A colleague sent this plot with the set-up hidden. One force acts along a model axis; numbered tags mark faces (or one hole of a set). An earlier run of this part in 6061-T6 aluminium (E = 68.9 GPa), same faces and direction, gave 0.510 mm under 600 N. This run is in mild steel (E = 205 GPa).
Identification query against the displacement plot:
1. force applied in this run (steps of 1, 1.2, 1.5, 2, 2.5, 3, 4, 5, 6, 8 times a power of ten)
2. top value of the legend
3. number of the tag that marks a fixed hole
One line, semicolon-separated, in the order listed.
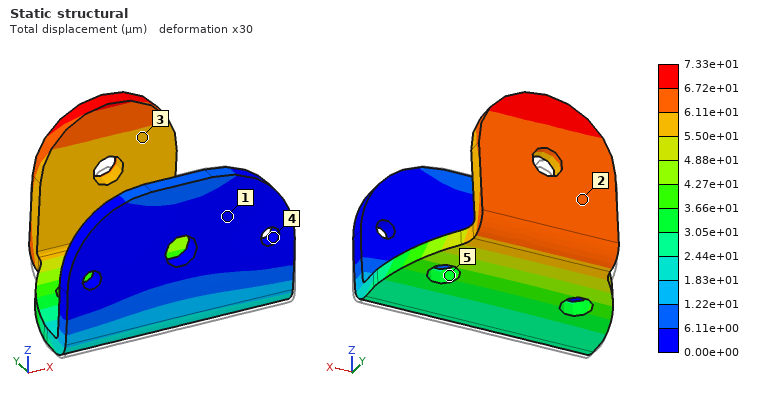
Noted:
250 N; 7.33e+01 µm; 4
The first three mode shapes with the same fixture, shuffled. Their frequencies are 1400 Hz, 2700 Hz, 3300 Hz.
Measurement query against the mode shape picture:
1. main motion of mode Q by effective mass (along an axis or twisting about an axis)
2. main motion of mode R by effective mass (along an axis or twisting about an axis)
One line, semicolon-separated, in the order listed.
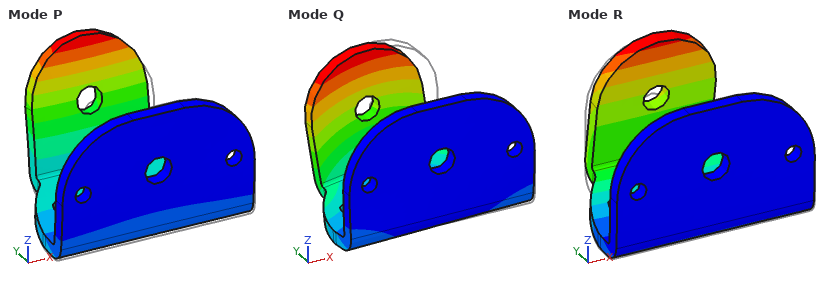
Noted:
along X; along Z
